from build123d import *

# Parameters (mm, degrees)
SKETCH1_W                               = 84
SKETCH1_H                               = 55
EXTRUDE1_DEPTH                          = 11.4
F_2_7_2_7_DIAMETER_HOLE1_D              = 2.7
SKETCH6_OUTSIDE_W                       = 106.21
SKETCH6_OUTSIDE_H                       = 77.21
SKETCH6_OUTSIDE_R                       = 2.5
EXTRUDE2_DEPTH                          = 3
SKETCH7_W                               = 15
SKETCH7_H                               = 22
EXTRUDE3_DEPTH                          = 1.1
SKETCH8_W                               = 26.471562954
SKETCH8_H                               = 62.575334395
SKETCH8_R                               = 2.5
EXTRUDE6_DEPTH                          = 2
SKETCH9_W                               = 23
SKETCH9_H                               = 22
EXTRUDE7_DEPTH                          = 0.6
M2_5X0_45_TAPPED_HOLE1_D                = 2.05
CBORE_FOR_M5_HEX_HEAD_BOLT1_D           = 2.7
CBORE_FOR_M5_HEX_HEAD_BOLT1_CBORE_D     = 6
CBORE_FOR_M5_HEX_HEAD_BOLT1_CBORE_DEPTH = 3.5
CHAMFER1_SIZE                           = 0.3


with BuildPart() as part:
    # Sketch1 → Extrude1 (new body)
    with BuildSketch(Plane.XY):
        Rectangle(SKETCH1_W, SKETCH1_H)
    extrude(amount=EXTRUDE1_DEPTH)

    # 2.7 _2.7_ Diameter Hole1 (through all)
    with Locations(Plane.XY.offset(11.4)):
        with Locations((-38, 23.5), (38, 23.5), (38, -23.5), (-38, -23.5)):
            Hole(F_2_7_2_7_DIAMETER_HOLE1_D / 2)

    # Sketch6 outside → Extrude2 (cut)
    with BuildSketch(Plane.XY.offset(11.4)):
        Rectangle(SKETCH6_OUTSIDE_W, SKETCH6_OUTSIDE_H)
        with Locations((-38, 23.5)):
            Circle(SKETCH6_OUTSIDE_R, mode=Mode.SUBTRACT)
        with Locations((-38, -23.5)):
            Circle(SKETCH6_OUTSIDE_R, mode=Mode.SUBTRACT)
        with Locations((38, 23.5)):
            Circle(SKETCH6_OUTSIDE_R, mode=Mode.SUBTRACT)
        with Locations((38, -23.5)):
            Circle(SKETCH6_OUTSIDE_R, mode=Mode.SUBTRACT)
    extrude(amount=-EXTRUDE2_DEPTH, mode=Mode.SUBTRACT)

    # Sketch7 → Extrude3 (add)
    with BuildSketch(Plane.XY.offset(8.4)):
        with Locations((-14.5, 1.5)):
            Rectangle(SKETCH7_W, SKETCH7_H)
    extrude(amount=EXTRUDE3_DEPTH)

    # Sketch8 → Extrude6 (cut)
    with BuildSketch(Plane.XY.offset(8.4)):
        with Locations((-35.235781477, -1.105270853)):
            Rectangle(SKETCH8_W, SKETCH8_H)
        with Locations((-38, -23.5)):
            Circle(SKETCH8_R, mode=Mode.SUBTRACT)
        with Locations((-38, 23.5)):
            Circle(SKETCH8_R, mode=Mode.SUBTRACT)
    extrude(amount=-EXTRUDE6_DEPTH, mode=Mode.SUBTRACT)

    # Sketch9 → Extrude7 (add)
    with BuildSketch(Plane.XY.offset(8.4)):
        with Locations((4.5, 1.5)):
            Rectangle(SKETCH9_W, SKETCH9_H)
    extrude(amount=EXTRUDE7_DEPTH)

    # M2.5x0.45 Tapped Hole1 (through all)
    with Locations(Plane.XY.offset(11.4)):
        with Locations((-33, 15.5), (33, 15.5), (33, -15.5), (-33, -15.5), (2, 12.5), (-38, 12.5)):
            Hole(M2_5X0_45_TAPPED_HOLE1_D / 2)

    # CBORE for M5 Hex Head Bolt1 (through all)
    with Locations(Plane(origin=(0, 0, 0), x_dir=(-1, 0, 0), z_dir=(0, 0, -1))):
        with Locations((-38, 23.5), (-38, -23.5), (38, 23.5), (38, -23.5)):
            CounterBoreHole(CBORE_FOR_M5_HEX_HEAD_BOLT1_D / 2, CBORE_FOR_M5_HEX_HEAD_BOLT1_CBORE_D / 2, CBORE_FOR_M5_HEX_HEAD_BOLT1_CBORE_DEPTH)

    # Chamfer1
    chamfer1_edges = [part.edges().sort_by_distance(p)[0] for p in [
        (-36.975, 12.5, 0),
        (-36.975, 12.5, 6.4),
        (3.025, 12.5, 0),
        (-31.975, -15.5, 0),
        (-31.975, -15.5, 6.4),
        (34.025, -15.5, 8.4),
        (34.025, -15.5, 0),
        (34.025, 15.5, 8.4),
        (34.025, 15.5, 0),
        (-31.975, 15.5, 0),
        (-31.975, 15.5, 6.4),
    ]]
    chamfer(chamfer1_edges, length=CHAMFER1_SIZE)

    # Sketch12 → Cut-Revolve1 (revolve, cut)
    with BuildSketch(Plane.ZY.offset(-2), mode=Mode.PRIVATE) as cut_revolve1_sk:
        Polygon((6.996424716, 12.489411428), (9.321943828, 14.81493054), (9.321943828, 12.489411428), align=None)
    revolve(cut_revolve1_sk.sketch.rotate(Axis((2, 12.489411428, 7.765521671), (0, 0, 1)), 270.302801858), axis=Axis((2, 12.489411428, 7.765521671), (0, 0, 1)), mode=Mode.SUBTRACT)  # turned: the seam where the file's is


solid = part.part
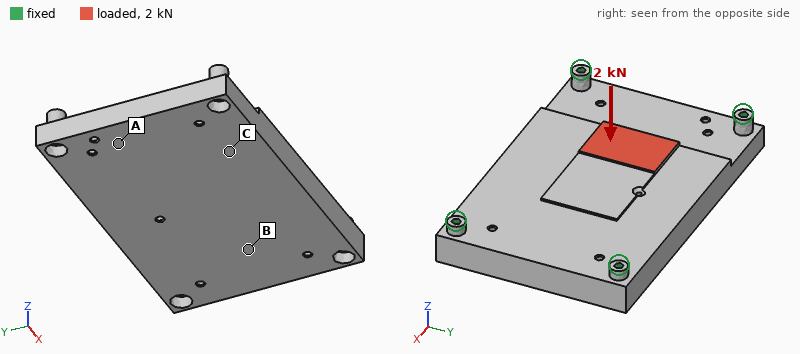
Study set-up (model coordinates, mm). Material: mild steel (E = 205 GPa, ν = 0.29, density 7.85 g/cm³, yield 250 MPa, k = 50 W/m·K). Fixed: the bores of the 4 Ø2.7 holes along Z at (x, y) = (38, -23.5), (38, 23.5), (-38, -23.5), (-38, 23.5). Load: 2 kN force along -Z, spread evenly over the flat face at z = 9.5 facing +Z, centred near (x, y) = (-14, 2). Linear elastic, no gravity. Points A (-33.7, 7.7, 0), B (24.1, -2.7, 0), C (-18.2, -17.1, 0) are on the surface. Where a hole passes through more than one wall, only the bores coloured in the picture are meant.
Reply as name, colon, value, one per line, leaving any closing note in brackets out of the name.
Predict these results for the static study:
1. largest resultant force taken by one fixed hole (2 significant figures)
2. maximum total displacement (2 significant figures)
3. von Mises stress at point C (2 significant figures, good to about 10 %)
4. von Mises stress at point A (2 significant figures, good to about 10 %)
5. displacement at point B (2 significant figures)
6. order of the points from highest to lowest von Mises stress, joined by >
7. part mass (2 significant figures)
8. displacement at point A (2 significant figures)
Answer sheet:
largest resultant force taken by one fixed hole: 930 N
maximum total displacement: 19 µm
von Mises stress at point C: 28 MPa
von Mises stress at point A: 21 MPa
displacement at point B: 7.7 µm
order of the points from highest to lowest von Mises stress, joined by >: C > A > B
part mass: 290 g
displacement at point A: 9.2 µm
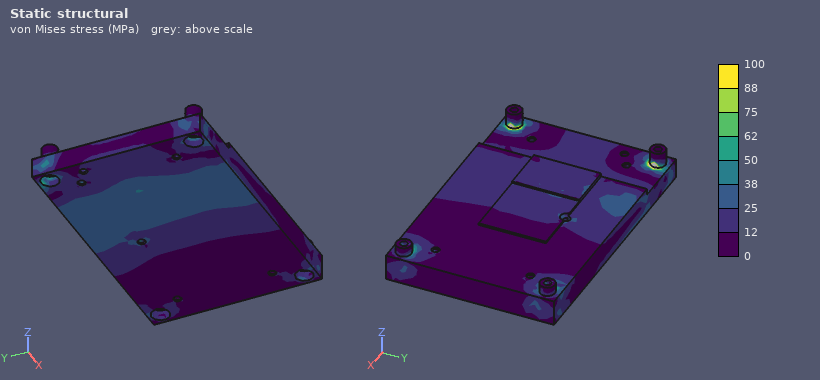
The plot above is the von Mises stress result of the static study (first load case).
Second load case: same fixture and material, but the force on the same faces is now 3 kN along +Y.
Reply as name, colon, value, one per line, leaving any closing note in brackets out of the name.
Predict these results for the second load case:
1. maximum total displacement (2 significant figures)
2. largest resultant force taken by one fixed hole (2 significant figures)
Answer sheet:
maximum total displacement: 7.9 µm
largest resultant force taken by one fixed hole: 970 N
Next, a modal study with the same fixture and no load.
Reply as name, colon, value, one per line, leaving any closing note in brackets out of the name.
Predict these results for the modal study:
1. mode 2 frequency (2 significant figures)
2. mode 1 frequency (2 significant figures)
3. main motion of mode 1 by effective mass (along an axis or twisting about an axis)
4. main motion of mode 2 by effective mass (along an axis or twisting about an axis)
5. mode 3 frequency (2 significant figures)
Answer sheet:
mode 2 frequency: 7200 Hz
mode 1 frequency: 4200 Hz
main motion of mode 1 by effective mass: along Z
main motion of mode 2 by effective mass: twisting about X
mode 3 frequency: 10 kHz
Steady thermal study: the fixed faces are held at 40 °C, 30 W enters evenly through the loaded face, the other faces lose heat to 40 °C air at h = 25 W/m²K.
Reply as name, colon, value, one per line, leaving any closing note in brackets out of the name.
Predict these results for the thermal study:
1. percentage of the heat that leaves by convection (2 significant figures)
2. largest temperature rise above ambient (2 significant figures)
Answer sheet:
percentage of the heat that leaves by convection: 19 %
largest temperature rise above ambient: 45 K
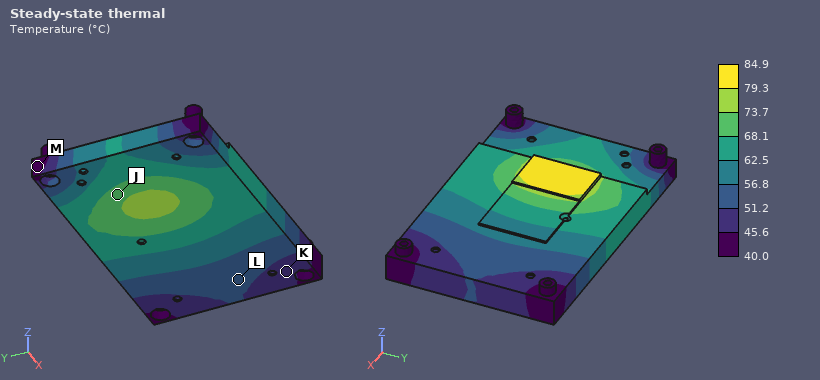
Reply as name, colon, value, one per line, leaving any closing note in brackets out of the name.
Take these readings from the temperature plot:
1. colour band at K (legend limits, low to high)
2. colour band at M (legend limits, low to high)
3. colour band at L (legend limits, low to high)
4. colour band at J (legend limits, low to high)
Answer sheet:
colour band at K: 45.6 to 51.2 °C
colour band at M: 40.0 to 45.6 °C
colour band at L: 51.2 to 56.8 °C
colour band at J: 68.1 to 73.7 °C
